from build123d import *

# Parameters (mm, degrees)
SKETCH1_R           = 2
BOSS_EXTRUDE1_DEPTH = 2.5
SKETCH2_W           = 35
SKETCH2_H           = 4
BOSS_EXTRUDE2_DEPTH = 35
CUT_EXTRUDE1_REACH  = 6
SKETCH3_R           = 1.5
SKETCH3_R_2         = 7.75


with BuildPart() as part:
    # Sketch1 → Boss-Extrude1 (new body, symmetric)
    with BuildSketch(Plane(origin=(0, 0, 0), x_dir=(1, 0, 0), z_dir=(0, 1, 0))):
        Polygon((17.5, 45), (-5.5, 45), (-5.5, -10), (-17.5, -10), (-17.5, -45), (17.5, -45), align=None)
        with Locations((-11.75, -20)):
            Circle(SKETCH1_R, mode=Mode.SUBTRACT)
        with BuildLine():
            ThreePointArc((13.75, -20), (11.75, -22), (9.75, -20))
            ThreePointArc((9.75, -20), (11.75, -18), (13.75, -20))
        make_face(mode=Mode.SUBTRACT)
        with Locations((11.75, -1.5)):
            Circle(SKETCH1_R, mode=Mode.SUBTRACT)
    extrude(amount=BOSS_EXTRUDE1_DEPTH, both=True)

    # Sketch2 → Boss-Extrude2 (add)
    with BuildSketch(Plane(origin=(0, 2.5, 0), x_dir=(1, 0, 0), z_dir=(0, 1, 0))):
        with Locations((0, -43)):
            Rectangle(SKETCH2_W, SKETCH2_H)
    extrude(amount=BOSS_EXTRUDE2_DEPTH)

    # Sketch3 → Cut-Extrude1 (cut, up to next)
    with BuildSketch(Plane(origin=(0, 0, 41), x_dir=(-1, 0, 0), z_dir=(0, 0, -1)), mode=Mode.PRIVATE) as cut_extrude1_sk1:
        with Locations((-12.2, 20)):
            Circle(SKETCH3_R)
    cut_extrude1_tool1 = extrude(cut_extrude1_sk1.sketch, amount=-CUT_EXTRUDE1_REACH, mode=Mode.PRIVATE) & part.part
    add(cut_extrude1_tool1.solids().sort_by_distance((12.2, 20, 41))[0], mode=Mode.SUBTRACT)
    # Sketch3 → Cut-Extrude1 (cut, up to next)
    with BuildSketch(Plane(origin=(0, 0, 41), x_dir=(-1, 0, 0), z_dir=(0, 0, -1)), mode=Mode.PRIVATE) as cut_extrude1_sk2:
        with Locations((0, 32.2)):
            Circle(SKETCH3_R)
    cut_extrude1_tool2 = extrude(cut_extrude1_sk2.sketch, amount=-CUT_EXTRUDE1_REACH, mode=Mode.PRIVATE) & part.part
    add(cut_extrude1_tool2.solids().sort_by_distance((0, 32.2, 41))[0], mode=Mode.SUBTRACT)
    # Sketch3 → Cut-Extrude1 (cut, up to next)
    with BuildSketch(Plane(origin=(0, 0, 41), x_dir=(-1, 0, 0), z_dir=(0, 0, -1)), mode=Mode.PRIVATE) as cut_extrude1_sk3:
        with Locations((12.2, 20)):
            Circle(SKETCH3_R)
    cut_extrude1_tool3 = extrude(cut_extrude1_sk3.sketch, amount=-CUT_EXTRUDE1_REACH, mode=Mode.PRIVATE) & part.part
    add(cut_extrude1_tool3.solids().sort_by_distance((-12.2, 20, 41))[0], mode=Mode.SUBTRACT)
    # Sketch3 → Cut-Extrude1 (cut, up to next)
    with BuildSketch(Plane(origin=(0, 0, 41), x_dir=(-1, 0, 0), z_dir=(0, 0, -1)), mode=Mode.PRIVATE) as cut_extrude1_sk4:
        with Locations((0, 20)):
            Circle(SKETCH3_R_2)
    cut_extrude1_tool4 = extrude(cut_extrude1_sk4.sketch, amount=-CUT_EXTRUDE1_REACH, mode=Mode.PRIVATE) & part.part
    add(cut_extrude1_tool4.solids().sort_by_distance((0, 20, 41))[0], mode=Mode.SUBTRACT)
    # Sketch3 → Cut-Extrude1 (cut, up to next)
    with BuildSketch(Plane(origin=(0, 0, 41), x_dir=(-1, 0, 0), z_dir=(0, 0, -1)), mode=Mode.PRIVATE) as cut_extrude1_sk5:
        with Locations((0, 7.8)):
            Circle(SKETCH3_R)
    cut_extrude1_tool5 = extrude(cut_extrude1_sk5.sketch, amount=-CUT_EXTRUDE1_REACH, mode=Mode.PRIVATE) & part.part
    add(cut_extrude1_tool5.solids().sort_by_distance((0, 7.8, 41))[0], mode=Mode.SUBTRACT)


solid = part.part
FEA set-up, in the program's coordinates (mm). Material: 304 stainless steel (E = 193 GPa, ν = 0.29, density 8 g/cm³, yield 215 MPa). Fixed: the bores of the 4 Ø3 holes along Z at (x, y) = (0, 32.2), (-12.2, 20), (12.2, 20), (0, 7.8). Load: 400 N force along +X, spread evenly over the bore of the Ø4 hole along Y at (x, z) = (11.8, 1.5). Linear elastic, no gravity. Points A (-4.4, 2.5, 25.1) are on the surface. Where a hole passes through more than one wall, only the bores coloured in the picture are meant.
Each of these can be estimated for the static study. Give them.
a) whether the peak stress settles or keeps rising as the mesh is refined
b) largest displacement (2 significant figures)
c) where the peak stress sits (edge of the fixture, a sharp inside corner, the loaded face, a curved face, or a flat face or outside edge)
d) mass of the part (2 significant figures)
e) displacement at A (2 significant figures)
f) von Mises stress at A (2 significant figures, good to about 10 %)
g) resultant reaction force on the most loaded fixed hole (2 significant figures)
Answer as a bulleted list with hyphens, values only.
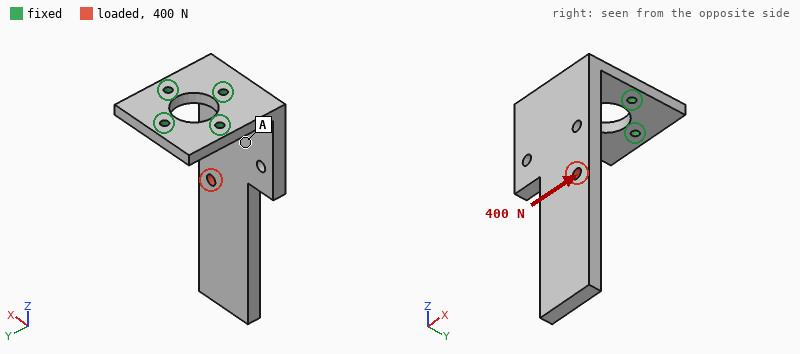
- keeps rising
- 0.19 mm
- edge of the fixture
- 130 g
- 0.039 mm
- 15 MPa
- 350 N
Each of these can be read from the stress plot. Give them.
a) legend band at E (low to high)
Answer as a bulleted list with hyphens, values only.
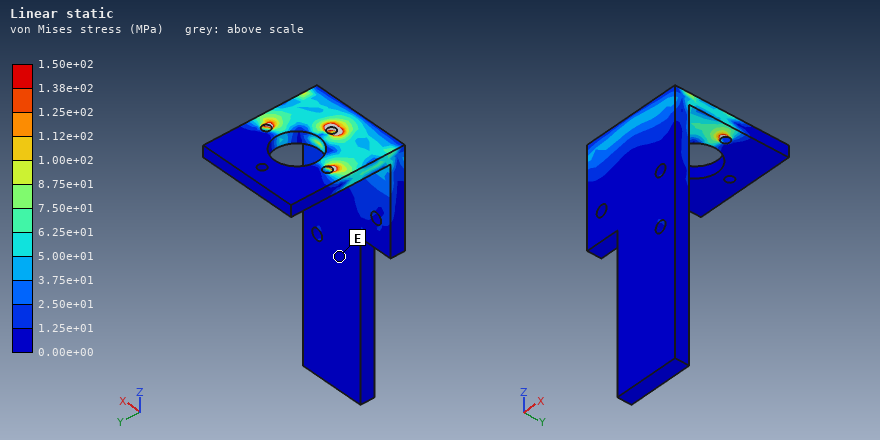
- 0.00e+00 to 1.25e+01 MPa
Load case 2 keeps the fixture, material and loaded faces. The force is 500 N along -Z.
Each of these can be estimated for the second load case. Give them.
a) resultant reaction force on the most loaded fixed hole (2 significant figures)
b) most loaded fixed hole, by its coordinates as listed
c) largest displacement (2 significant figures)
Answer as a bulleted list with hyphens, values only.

- 580 N
- (0, 7.8)
- 93 µm
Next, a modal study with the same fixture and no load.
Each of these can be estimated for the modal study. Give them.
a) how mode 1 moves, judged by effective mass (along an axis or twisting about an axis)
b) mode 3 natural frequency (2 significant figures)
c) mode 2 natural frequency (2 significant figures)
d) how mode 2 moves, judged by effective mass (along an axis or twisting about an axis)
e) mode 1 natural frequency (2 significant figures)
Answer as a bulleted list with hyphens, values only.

- along Y
- 2600 Hz
- 940 Hz
- along X
- 460 Hz
